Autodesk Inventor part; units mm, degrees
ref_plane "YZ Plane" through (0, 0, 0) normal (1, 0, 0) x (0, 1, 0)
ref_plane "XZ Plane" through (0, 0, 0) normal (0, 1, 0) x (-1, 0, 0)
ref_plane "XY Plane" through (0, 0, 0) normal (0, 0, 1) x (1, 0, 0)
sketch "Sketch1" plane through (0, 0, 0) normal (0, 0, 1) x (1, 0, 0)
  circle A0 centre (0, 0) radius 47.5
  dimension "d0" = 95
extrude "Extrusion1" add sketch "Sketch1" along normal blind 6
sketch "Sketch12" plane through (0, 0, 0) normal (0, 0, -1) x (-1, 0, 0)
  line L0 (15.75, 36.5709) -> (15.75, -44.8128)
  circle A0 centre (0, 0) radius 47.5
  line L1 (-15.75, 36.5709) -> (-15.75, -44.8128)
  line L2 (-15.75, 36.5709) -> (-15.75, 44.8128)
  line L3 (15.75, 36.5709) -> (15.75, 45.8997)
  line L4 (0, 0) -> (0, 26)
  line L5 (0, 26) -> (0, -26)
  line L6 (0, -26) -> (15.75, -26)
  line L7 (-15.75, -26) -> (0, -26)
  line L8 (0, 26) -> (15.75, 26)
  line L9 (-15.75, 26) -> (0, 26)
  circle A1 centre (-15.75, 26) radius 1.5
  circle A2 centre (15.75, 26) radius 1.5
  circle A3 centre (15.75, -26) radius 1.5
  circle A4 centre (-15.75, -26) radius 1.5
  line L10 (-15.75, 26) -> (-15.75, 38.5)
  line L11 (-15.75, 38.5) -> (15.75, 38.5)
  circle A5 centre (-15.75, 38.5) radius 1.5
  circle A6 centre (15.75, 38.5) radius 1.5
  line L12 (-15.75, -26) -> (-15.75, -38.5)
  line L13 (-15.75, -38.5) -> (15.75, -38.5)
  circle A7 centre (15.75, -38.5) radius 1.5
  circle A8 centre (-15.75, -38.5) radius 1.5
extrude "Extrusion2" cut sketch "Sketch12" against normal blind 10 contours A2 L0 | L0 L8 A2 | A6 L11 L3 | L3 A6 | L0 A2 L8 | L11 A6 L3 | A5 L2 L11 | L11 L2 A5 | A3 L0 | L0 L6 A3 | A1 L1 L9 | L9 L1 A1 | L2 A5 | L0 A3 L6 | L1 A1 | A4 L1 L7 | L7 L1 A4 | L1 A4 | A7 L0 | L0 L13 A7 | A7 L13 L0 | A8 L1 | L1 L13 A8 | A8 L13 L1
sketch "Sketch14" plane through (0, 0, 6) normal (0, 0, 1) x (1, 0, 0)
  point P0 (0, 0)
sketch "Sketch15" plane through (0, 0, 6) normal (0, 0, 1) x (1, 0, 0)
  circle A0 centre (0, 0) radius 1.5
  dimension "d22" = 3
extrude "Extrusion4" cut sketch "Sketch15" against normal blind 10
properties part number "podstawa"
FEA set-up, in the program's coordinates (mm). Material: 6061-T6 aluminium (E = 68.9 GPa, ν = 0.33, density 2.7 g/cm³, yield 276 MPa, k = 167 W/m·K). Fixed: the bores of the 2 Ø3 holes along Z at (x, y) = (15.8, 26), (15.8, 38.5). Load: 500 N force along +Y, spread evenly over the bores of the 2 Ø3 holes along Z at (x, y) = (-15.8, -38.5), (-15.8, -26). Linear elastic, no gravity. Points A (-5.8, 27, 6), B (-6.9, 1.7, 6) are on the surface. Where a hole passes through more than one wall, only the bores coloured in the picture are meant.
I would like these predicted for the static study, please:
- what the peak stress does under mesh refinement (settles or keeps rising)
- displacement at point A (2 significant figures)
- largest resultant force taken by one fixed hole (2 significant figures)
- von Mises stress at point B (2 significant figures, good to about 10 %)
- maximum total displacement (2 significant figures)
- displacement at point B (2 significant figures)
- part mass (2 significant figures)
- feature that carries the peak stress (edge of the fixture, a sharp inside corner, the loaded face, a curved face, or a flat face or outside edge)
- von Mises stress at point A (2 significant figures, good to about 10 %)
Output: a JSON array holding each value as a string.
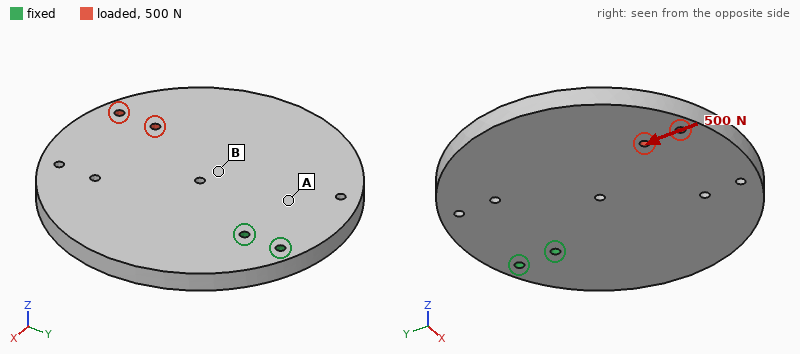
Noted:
["keeps rising", "8.0 µm", "1.1 kN", "2.2 MPa", "30 µm", "13 µm", "110 g", "edge of the fixture", "3.9 MPa"]
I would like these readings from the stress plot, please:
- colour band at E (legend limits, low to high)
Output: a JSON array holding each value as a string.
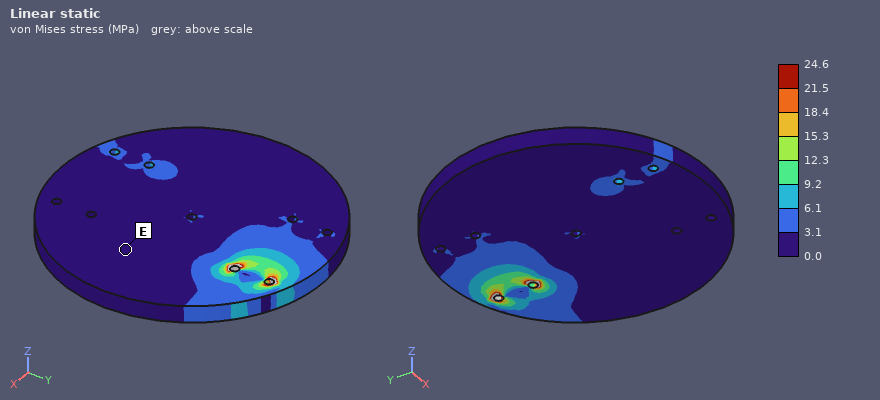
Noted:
["0.0 to 3.1 MPa"]
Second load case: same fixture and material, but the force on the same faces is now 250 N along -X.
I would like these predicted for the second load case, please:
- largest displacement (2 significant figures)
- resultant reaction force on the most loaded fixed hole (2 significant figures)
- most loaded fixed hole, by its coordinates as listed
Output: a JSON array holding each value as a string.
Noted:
["29 µm", "1.2 kN", "(15.8, 26)"]
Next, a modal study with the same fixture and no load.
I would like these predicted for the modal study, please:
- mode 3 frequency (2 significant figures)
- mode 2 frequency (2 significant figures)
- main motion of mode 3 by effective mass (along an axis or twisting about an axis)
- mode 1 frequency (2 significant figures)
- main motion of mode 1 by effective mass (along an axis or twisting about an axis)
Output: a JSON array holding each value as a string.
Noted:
["2100 Hz", "1200 Hz", "along X", "730 Hz", "along Z"]
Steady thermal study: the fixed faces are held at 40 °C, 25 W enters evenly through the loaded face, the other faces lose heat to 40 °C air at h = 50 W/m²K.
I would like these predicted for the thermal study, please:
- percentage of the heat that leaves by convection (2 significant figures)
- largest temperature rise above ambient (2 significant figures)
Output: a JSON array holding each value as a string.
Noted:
["36 %", "27 K"]
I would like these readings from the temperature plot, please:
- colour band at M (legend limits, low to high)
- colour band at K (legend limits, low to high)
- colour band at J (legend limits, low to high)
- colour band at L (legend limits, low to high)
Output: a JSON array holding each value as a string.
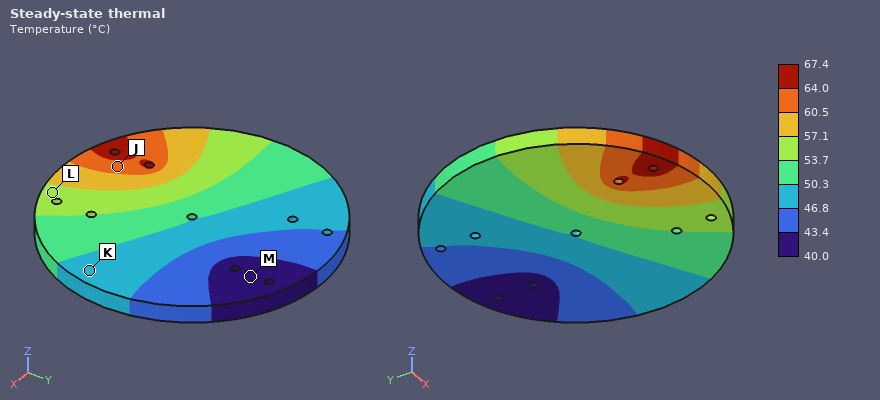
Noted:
["40.0 to 43.4 °C", "46.8 to 50.3 °C", "60.5 to 64.0 °C", "53.7 to 57.1 °C"]
